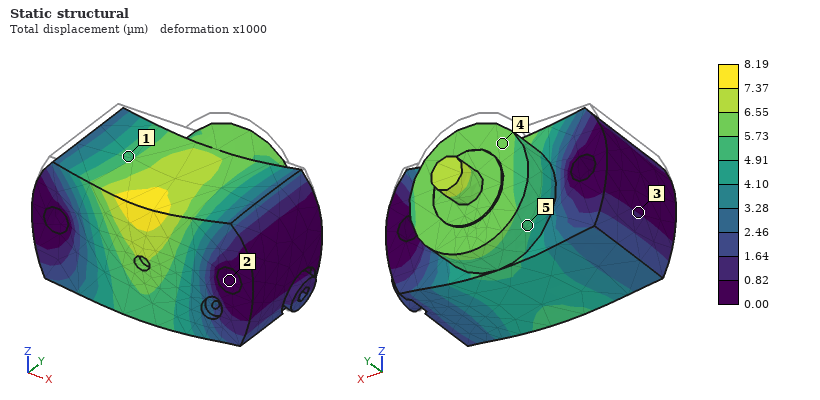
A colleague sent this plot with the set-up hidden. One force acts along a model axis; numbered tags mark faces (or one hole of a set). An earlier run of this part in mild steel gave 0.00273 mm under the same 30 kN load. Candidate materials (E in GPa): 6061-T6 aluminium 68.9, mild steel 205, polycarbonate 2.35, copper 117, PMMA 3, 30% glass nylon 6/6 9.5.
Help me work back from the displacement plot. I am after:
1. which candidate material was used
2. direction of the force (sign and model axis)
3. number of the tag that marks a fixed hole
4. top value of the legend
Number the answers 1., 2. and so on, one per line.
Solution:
1. 6061-T6 aluminium
2. -Z
3. 2
4. 8.19 µm
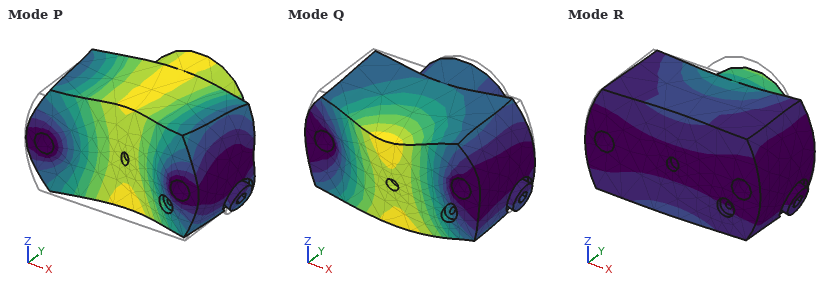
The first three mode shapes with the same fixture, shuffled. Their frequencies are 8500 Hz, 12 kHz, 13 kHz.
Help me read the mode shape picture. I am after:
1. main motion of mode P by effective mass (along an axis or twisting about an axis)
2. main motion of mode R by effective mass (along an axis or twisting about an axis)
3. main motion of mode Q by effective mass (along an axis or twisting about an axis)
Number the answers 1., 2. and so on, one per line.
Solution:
1. along Y
2. along Z
3. along Z
